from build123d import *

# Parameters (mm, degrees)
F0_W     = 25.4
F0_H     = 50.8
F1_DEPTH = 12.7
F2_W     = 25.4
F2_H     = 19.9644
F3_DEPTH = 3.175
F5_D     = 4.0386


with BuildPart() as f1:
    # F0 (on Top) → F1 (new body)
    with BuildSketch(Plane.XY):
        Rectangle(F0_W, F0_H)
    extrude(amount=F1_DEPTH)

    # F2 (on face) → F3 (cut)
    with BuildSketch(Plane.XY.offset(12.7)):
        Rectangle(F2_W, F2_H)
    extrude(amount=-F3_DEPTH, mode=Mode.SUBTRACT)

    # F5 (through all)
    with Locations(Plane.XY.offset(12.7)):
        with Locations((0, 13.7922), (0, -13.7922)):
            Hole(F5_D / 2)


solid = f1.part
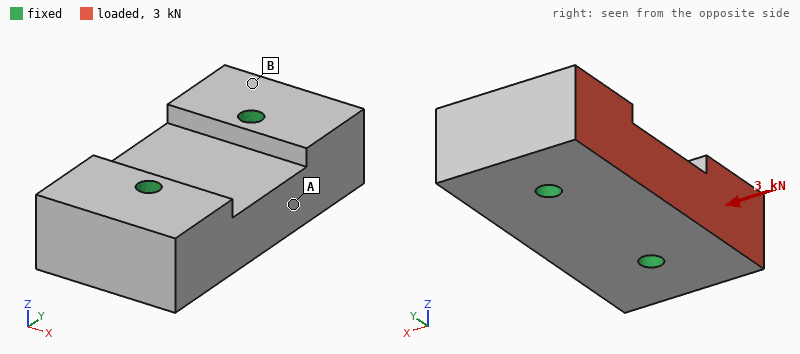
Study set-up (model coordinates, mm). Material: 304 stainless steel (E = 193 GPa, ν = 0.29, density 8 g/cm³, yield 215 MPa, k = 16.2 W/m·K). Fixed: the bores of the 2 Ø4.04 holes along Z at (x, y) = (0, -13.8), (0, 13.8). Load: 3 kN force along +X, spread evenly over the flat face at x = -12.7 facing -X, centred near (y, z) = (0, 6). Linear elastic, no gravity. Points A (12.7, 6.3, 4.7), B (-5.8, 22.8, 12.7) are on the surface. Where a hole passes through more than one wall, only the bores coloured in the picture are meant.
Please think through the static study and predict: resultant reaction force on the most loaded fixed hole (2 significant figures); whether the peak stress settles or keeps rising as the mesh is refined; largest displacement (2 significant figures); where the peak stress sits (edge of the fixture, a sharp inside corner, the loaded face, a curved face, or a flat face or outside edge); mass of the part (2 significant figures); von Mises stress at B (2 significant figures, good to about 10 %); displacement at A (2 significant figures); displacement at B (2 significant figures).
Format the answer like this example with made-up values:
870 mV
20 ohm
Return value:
1.5 kN
keeps rising
0.81 µm
edge of the fixture
120 g
4.0 MPa
0.19 µm
0.48 µm
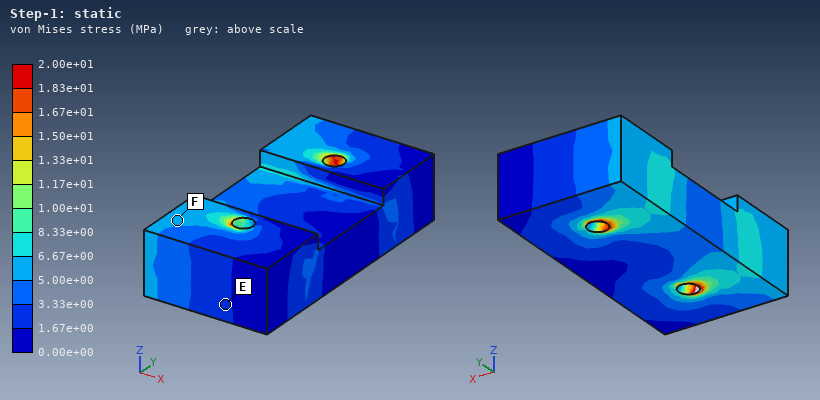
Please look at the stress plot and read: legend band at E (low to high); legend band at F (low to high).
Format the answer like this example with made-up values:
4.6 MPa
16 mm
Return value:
1.67e+00 to 3.33e+00 MPa
5.00e+00 to 6.67e+00 MPa
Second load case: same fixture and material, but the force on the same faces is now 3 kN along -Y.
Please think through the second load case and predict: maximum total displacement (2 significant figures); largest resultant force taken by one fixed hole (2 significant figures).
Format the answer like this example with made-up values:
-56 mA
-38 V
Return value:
2.8 µm
1.9 kN
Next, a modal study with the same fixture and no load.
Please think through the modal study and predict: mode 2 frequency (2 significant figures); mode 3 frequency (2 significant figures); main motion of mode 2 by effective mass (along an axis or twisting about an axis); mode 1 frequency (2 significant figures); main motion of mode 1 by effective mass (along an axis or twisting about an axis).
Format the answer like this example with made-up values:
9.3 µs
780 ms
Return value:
31 kHz
33 kHz
twisting about Z
28 kHz
twisting about Y
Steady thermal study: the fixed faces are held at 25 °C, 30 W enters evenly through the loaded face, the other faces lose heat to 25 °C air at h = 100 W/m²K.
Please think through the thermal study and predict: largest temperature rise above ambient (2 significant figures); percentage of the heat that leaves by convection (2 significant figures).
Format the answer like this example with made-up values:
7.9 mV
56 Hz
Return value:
45 K
18 %
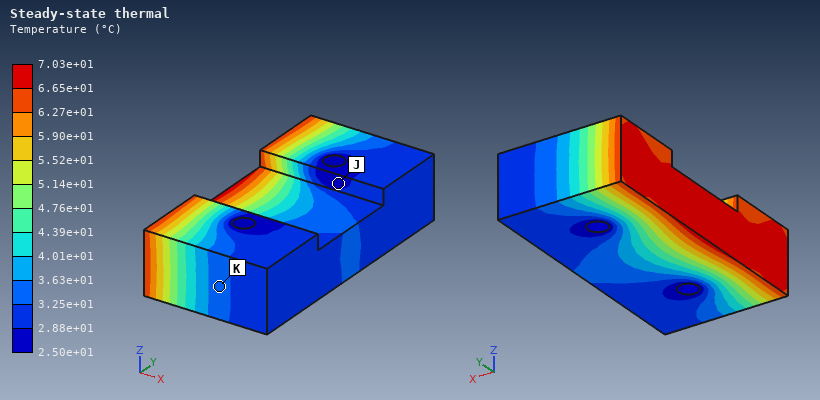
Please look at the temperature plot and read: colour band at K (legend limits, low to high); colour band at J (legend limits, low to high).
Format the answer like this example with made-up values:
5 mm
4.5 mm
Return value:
3.25e+01 to 3.63e+01 °C
2.50e+01 to 2.88e+01 °C
